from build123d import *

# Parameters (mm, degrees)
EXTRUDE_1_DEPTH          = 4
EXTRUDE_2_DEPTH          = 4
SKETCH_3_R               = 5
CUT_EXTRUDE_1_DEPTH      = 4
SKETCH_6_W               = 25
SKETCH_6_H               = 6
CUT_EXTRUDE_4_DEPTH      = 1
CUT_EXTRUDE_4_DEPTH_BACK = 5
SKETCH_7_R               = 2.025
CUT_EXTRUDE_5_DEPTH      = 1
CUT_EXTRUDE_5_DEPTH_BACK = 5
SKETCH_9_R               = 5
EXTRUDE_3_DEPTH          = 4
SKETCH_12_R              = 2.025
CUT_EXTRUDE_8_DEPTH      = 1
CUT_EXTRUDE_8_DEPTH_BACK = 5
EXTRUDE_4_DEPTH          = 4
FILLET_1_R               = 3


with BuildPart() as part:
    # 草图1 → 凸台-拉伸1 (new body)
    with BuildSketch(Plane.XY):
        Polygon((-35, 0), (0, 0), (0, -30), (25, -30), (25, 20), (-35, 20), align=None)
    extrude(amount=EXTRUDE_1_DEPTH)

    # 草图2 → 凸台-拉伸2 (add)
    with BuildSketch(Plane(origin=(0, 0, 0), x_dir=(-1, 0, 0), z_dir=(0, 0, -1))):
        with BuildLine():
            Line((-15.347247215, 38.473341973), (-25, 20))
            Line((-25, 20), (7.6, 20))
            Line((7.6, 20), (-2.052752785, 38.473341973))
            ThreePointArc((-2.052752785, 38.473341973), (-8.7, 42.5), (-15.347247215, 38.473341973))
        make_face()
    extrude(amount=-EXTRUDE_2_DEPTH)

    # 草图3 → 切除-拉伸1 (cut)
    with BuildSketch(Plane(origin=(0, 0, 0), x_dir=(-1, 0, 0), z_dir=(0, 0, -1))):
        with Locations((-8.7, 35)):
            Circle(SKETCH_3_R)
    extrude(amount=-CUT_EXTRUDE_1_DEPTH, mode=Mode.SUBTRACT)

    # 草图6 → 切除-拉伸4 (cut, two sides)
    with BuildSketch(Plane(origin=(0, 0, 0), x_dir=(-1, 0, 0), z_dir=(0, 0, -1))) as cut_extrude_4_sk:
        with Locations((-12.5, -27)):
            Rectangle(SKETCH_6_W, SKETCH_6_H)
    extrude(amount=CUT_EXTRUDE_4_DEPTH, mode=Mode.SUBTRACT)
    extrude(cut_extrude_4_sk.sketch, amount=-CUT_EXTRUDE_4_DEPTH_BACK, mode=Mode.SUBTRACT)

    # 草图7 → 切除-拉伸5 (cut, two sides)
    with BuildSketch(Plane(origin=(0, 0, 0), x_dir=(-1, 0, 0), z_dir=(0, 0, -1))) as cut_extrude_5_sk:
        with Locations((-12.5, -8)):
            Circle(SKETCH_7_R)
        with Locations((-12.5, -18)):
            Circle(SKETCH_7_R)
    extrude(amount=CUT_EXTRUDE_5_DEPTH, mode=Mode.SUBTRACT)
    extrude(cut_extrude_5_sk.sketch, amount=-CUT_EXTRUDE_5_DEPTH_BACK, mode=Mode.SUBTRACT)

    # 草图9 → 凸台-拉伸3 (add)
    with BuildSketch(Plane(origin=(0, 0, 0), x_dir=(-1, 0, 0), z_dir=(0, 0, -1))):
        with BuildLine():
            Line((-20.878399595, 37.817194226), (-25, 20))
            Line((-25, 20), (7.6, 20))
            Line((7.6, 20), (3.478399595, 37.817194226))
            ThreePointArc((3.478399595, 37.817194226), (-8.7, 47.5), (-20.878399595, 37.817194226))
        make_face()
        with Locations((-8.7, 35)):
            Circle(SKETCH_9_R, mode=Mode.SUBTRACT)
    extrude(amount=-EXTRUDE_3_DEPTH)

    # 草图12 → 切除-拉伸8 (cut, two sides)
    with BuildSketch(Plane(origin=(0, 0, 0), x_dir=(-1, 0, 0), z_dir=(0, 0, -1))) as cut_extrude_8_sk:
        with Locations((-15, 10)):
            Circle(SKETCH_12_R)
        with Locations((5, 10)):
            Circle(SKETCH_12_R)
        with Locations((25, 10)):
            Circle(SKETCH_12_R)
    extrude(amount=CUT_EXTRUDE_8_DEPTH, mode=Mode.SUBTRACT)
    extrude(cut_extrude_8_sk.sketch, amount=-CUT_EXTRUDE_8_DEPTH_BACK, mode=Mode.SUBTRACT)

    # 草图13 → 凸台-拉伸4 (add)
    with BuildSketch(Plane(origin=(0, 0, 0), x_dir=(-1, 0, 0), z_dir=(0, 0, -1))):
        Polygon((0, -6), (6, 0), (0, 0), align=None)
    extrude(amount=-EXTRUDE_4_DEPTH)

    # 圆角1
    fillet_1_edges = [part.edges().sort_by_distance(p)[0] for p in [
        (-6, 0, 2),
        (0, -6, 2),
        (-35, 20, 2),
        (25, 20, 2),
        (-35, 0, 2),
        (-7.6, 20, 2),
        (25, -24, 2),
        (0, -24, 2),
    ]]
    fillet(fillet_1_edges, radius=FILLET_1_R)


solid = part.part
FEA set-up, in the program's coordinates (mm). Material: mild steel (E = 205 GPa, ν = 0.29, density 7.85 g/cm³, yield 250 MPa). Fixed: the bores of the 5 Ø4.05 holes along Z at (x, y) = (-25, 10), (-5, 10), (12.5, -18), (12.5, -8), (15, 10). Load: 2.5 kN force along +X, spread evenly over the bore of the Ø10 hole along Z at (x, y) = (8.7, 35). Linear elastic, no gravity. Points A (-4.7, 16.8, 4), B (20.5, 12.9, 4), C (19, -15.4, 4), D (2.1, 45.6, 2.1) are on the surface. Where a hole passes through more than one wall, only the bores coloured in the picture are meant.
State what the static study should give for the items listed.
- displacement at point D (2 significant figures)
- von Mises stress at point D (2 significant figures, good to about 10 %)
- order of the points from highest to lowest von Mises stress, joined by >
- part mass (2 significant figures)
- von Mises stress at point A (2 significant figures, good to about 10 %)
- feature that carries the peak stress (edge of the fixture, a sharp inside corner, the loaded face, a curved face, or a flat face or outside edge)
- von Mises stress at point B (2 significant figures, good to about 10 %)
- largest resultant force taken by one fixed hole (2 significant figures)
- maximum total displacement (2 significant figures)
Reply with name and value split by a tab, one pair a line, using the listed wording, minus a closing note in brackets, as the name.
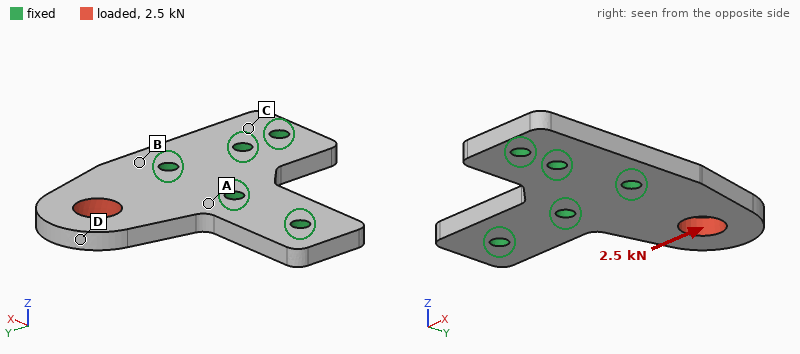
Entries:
displacement at point D	19 µm
von Mises stress at point D	25 MPa
order of the points from highest to lowest von Mises stress, joined by >	A > B > D > C
part mass	74 g
von Mises stress at point A	47 MPa
feature that carries the peak stress	a curved face
von Mises stress at point B	36 MPa
largest resultant force taken by one fixed hole	2.2 kN
maximum total displacement	19 µm
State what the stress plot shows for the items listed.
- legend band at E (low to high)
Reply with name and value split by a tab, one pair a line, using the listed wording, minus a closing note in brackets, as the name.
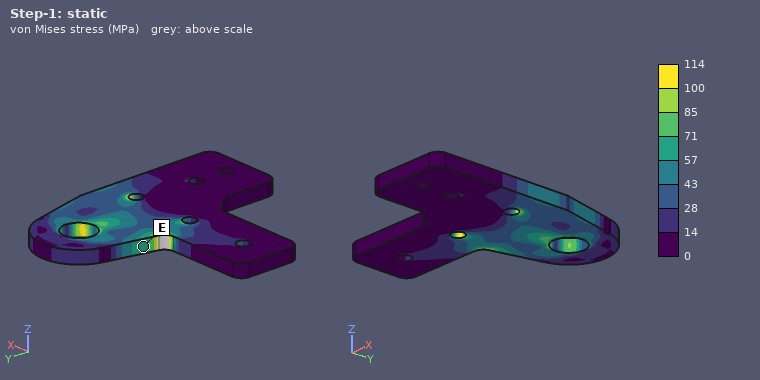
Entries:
legend band at E	57 to 71 MPa
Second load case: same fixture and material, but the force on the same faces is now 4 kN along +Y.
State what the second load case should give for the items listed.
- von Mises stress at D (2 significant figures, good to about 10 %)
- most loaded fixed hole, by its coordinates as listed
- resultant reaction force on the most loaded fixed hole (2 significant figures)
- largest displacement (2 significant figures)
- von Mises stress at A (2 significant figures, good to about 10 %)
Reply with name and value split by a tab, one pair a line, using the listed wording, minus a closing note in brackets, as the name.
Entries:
von Mises stress at D	27 MPa
most loaded fixed hole, by its coordinates as listed	(15, 10)
resultant reaction force on the most loaded fixed hole	2.2 kN
largest displacement	7.8 µm
von Mises stress at A	30 MPa
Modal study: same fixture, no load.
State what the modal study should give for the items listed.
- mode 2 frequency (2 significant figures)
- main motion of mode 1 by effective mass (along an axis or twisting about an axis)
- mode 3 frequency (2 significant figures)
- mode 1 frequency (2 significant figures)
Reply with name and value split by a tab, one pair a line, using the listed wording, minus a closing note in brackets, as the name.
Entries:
mode 2 frequency	9500 Hz
main motion of mode 1 by effective mass	along Z
mode 3 frequency	15 kHz
mode 1 frequency	3300 Hz
